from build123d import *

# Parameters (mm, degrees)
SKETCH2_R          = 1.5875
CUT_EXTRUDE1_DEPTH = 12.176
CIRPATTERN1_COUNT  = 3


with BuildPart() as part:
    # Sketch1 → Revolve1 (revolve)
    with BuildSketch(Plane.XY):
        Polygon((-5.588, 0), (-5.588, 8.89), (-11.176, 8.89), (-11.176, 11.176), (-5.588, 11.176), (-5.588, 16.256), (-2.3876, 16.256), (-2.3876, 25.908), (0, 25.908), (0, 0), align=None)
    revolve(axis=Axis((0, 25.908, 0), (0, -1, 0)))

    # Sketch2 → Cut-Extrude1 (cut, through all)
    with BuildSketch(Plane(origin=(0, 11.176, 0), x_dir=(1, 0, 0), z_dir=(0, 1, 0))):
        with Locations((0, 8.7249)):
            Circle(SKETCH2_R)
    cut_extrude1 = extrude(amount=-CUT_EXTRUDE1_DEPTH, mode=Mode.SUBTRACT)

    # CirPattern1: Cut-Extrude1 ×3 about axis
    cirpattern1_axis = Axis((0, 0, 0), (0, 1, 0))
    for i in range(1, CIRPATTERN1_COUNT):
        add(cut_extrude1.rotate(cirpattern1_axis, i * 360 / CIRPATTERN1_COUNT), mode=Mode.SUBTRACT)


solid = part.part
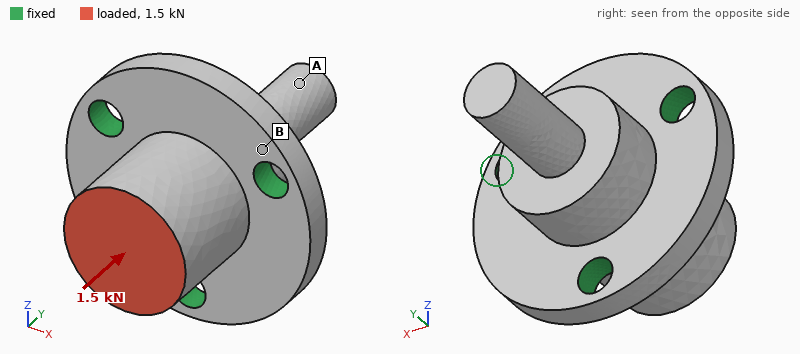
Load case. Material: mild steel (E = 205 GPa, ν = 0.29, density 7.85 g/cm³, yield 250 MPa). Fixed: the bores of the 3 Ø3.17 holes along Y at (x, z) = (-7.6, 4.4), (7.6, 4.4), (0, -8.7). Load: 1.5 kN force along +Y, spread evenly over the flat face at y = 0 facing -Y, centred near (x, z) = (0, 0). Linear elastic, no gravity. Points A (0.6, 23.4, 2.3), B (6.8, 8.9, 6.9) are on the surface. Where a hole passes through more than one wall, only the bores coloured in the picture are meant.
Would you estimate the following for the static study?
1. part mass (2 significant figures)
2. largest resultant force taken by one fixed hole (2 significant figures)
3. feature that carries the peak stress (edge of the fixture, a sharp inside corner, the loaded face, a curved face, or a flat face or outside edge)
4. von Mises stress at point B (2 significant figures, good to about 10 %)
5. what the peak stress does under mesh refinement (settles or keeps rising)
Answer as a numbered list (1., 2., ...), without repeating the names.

1. 19 g
2. 500 N
3. edge of the fixture
4. 21 MPa
5. keeps rising
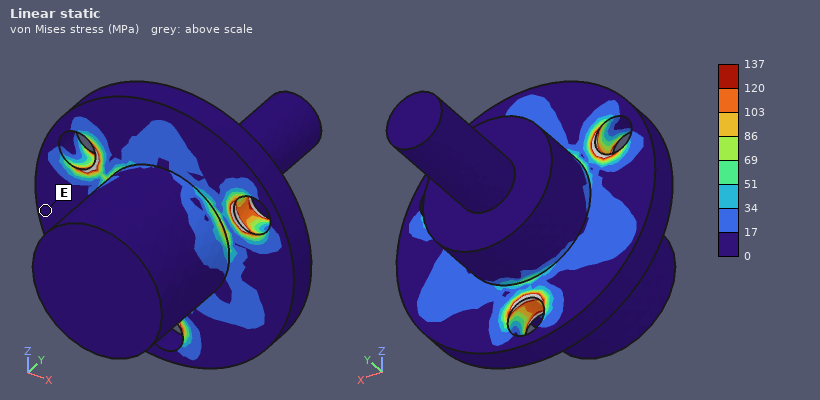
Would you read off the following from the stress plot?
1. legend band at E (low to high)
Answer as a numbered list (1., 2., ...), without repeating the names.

1. 0 to 17 MPa
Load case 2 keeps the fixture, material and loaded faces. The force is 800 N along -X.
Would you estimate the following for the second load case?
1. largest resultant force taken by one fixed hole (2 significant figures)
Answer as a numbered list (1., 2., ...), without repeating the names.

1. 670 N
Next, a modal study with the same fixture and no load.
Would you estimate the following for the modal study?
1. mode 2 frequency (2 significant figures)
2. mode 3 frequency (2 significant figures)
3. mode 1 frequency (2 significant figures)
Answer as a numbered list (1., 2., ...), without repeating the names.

1. 22 kHz
2. 33 kHz
3. 22 kHz
